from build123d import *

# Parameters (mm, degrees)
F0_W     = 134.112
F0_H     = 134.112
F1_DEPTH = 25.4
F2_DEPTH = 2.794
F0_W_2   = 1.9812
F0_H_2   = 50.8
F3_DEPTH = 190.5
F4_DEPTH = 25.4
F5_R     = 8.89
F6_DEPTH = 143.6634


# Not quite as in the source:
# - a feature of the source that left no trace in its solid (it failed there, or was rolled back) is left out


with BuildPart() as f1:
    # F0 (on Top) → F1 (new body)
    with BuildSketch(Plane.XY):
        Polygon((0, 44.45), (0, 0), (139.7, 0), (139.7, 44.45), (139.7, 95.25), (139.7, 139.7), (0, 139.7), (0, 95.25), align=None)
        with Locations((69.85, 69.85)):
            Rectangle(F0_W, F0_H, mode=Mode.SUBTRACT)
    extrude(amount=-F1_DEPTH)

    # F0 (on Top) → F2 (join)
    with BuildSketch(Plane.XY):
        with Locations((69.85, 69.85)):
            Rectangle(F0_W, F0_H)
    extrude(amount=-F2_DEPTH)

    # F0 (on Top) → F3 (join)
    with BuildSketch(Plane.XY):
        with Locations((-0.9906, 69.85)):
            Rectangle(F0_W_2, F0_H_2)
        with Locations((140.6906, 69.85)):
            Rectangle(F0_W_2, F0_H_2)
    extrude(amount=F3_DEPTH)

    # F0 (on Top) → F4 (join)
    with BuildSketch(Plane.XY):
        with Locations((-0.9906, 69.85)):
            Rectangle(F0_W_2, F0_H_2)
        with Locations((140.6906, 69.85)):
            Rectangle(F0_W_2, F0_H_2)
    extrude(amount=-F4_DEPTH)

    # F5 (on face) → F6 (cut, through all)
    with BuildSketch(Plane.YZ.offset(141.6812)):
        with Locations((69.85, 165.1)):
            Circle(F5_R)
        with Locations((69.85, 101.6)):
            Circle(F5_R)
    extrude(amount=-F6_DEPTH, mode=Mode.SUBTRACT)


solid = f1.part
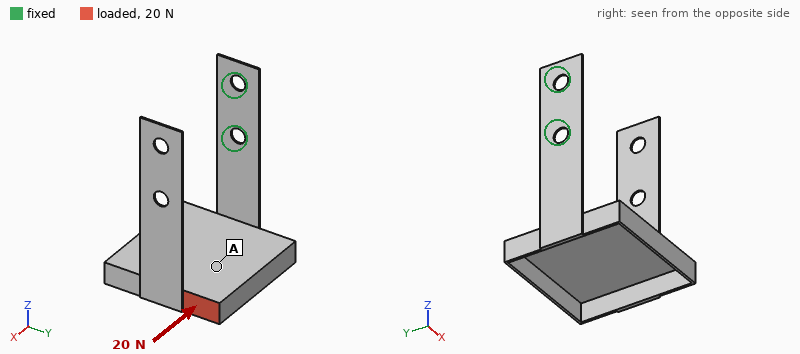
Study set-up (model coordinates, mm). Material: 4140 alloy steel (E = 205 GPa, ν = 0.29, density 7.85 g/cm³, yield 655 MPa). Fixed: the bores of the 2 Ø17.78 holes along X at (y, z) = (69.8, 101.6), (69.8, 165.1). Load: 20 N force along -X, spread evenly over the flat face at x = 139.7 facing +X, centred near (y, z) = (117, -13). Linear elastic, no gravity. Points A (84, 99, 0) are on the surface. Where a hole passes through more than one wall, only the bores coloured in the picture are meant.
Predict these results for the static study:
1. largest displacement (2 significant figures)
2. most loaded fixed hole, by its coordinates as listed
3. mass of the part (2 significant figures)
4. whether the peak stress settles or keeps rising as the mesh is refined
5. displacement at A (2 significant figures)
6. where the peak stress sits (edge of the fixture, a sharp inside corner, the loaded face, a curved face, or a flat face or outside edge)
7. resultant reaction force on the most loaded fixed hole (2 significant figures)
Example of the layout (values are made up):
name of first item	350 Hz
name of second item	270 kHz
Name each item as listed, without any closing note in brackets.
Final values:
largest displacement	3.5 mm
most loaded fixed hole, by its coordinates as listed	(69.8, 101.6)
mass of the part	1.0 kg
whether the peak stress settles or keeps rising as the mesh is refined	keeps rising
displacement at A	2.0 mm
where the peak stress sits	edge of the fixture
resultant reaction force on the most loaded fixed hole	20 N
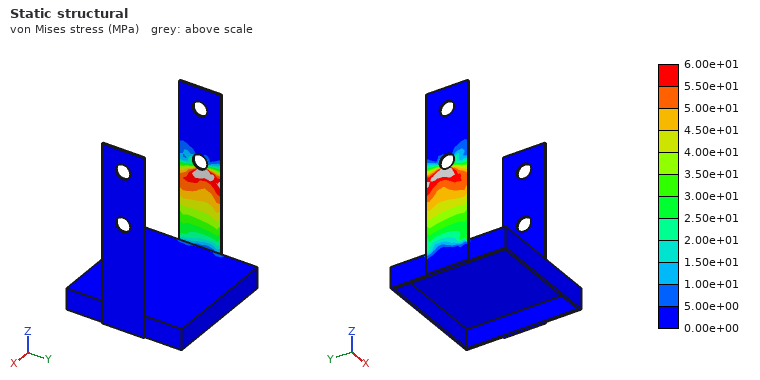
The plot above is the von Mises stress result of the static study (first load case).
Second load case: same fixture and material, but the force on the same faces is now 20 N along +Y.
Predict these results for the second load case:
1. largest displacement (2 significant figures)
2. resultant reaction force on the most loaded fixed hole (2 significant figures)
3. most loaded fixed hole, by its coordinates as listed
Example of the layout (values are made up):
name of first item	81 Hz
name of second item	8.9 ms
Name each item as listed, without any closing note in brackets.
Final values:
largest displacement	3.4 mm
resultant reaction force on the most loaded fixed hole	35 N
most loaded fixed hole, by its coordinates as listed	(69.8, 101.6)
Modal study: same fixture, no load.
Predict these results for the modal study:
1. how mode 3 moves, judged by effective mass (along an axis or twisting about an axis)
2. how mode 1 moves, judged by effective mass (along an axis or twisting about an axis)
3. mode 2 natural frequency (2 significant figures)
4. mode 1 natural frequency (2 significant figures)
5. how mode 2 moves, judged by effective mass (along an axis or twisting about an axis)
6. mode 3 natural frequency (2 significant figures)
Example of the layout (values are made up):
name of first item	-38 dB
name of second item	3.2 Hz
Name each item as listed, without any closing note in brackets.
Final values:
how mode 3 moves, judged by effective mass	along X
how mode 1 moves, judged by effective mass	along Z
mode 2 natural frequency	18 Hz
mode 1 natural frequency	13 Hz
how mode 2 moves, judged by effective mass	along Y
mode 3 natural frequency	41 Hz
